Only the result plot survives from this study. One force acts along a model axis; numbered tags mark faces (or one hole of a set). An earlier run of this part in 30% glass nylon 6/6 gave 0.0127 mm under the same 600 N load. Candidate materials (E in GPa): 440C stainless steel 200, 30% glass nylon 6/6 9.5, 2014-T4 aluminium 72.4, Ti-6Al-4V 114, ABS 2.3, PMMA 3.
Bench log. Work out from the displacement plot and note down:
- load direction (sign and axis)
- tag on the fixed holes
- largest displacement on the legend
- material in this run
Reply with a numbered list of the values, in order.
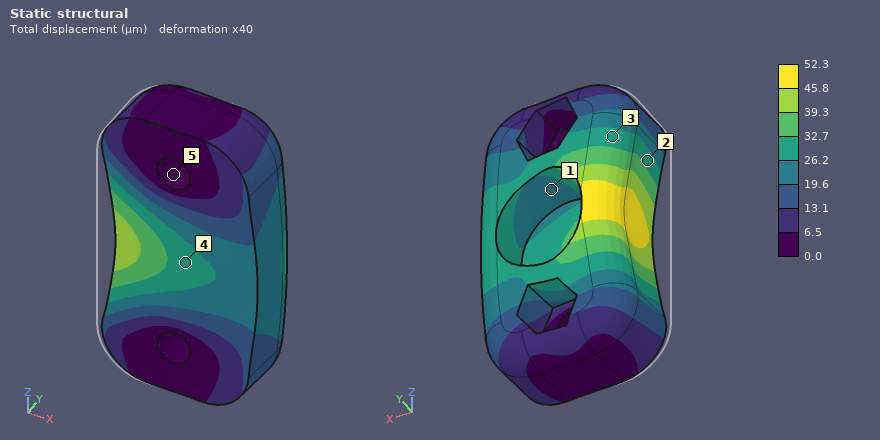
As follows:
1. +X
2. 5
3. 52.3 µm
4. ABS
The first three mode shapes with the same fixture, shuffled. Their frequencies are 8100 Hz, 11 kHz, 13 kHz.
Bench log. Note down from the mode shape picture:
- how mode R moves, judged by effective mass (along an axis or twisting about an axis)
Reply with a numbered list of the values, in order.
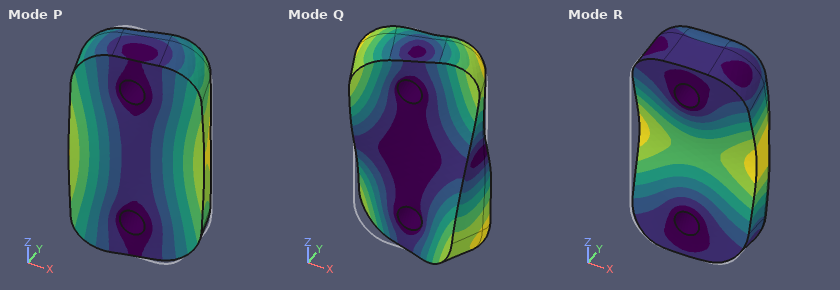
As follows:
1. along Y
